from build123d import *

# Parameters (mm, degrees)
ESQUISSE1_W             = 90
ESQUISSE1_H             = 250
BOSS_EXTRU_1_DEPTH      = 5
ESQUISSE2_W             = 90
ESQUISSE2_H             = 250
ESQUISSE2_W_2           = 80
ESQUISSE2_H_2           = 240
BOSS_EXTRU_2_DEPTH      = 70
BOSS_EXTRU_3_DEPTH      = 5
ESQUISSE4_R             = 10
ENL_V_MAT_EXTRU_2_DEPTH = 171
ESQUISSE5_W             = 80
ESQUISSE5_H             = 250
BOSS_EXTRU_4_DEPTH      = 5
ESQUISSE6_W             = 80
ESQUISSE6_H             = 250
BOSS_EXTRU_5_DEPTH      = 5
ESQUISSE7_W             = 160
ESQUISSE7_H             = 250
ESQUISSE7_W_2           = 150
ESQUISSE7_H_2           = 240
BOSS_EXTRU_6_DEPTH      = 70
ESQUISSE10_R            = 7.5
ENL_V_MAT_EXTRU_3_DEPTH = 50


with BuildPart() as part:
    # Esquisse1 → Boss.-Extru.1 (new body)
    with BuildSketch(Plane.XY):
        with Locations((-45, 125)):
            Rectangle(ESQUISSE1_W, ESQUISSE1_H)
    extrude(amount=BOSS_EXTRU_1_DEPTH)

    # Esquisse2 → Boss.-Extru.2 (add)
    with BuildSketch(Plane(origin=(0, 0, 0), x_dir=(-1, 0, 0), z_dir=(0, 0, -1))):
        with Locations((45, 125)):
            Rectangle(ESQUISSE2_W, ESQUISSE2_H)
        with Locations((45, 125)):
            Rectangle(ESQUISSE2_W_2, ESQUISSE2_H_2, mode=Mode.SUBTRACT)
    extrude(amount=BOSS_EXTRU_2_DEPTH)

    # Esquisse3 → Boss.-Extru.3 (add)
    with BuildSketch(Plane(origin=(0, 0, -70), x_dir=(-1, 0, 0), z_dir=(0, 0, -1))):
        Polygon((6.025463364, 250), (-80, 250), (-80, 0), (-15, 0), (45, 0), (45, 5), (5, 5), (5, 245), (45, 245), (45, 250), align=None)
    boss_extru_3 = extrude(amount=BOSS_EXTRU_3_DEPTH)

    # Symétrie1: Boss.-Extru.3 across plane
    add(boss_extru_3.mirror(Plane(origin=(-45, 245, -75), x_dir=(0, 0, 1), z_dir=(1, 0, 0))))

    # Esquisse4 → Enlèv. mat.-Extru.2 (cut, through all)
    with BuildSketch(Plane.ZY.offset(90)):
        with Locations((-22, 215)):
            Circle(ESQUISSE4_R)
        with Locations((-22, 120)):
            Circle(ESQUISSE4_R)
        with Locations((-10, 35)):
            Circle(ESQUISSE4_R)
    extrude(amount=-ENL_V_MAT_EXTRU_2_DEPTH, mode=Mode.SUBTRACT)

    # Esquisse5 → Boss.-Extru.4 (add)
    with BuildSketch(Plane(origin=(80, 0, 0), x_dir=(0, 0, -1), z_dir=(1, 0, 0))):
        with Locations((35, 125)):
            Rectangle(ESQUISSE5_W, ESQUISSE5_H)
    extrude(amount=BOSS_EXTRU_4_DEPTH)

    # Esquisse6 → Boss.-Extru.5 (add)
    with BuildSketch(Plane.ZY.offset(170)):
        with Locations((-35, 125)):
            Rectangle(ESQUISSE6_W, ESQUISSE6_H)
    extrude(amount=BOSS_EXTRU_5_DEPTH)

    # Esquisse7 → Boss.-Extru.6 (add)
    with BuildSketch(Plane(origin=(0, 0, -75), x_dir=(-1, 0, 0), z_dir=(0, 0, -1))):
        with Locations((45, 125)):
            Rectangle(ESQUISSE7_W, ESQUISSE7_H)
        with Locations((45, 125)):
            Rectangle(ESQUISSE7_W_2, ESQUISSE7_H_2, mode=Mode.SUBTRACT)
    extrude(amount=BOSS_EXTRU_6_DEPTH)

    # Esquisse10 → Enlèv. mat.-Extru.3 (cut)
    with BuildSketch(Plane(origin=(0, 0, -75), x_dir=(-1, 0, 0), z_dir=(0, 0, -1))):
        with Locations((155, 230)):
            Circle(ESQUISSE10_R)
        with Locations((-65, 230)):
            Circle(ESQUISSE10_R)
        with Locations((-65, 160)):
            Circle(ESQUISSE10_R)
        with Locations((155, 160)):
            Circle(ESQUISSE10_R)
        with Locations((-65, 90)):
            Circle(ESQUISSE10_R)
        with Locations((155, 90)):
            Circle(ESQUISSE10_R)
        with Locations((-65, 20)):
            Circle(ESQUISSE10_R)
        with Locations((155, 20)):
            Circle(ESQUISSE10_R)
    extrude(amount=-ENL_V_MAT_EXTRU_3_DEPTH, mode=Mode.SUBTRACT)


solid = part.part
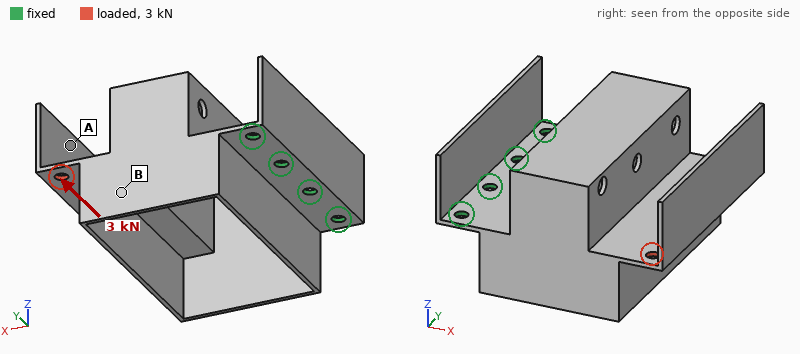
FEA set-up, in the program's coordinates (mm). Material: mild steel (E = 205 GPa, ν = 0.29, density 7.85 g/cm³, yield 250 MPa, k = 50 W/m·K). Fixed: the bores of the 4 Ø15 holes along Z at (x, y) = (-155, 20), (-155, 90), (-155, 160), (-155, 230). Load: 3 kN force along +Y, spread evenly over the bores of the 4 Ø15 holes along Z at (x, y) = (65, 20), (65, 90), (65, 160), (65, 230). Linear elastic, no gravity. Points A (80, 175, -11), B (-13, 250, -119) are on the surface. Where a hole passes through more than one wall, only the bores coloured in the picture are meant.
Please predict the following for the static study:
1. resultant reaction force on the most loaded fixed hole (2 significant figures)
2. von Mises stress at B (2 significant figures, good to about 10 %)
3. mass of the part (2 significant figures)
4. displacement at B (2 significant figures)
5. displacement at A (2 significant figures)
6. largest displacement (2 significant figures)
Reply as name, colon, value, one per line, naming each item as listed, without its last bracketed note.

resultant reaction force on the most loaded fixed hole: 3.0 kN
von Mises stress at B: 38 MPa
mass of the part: 8.0 kg
displacement at B: 0.57 mm
displacement at A: 0.25 mm
largest displacement: 0.83 mm
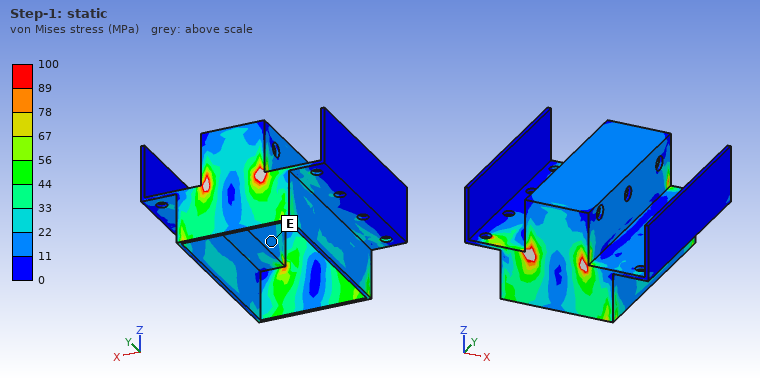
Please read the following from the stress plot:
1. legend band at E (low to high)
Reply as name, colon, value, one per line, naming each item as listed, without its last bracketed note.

legend band at E: 11 to 22 MPa
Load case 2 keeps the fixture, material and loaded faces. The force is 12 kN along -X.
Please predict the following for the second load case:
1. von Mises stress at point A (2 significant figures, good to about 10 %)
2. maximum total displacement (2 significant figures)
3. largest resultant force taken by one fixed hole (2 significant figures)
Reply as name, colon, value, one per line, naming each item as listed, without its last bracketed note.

von Mises stress at point A: 4.4 MPa
maximum total displacement: 0.20 mm
largest resultant force taken by one fixed hole: 5.9 kN
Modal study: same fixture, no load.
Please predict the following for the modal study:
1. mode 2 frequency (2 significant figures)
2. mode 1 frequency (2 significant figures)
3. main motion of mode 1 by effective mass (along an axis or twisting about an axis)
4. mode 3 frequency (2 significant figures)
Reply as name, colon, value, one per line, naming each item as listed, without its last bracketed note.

mode 2 frequency: 170 Hz
mode 1 frequency: 56 Hz
main motion of mode 1 by effective mass: along Z
mode 3 frequency: 320 Hz
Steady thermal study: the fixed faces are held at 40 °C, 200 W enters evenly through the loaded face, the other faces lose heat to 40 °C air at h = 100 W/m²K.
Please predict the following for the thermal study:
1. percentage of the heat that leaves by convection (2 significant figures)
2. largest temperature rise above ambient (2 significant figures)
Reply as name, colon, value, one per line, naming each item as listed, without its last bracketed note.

percentage of the heat that leaves by convection: 100 %
largest temperature rise above ambient: 75 K
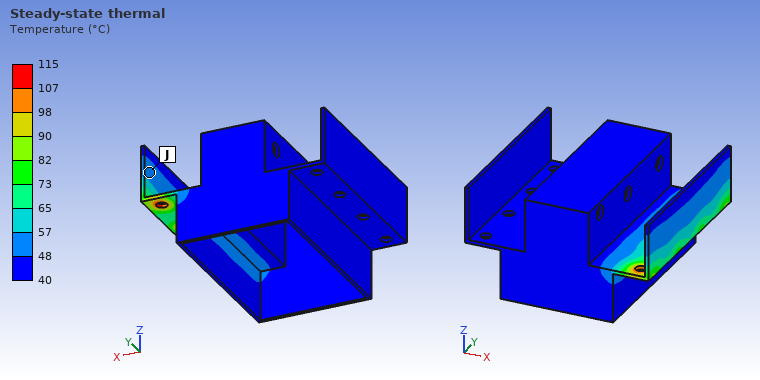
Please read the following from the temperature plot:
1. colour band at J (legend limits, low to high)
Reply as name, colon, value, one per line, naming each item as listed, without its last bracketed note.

colour band at J: 48 to 57 °C
